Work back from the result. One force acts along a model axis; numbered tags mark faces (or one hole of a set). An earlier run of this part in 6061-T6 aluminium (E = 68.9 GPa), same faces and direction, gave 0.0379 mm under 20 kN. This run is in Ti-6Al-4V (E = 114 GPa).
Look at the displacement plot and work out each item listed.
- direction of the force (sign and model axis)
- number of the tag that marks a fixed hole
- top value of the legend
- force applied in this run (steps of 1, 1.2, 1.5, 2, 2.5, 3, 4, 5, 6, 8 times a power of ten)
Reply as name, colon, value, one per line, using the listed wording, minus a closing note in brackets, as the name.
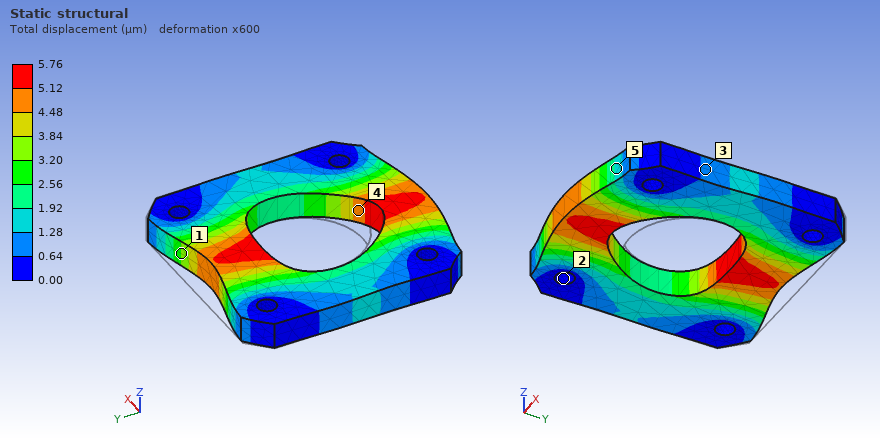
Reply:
direction of the force: -Y
number of the tag that marks a fixed hole: 2
top value of the legend: 5.76 µm
force applied in this run: 5 kN
